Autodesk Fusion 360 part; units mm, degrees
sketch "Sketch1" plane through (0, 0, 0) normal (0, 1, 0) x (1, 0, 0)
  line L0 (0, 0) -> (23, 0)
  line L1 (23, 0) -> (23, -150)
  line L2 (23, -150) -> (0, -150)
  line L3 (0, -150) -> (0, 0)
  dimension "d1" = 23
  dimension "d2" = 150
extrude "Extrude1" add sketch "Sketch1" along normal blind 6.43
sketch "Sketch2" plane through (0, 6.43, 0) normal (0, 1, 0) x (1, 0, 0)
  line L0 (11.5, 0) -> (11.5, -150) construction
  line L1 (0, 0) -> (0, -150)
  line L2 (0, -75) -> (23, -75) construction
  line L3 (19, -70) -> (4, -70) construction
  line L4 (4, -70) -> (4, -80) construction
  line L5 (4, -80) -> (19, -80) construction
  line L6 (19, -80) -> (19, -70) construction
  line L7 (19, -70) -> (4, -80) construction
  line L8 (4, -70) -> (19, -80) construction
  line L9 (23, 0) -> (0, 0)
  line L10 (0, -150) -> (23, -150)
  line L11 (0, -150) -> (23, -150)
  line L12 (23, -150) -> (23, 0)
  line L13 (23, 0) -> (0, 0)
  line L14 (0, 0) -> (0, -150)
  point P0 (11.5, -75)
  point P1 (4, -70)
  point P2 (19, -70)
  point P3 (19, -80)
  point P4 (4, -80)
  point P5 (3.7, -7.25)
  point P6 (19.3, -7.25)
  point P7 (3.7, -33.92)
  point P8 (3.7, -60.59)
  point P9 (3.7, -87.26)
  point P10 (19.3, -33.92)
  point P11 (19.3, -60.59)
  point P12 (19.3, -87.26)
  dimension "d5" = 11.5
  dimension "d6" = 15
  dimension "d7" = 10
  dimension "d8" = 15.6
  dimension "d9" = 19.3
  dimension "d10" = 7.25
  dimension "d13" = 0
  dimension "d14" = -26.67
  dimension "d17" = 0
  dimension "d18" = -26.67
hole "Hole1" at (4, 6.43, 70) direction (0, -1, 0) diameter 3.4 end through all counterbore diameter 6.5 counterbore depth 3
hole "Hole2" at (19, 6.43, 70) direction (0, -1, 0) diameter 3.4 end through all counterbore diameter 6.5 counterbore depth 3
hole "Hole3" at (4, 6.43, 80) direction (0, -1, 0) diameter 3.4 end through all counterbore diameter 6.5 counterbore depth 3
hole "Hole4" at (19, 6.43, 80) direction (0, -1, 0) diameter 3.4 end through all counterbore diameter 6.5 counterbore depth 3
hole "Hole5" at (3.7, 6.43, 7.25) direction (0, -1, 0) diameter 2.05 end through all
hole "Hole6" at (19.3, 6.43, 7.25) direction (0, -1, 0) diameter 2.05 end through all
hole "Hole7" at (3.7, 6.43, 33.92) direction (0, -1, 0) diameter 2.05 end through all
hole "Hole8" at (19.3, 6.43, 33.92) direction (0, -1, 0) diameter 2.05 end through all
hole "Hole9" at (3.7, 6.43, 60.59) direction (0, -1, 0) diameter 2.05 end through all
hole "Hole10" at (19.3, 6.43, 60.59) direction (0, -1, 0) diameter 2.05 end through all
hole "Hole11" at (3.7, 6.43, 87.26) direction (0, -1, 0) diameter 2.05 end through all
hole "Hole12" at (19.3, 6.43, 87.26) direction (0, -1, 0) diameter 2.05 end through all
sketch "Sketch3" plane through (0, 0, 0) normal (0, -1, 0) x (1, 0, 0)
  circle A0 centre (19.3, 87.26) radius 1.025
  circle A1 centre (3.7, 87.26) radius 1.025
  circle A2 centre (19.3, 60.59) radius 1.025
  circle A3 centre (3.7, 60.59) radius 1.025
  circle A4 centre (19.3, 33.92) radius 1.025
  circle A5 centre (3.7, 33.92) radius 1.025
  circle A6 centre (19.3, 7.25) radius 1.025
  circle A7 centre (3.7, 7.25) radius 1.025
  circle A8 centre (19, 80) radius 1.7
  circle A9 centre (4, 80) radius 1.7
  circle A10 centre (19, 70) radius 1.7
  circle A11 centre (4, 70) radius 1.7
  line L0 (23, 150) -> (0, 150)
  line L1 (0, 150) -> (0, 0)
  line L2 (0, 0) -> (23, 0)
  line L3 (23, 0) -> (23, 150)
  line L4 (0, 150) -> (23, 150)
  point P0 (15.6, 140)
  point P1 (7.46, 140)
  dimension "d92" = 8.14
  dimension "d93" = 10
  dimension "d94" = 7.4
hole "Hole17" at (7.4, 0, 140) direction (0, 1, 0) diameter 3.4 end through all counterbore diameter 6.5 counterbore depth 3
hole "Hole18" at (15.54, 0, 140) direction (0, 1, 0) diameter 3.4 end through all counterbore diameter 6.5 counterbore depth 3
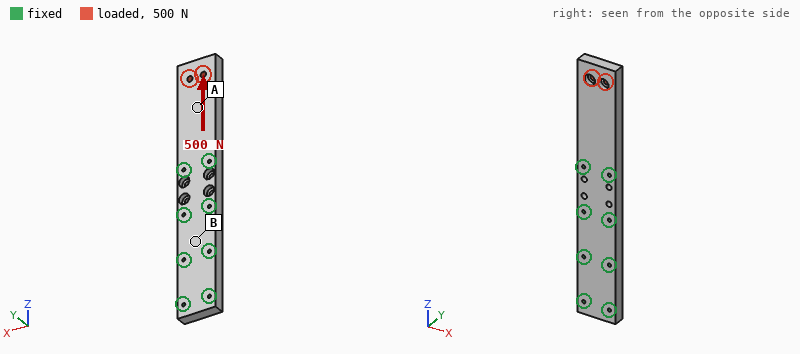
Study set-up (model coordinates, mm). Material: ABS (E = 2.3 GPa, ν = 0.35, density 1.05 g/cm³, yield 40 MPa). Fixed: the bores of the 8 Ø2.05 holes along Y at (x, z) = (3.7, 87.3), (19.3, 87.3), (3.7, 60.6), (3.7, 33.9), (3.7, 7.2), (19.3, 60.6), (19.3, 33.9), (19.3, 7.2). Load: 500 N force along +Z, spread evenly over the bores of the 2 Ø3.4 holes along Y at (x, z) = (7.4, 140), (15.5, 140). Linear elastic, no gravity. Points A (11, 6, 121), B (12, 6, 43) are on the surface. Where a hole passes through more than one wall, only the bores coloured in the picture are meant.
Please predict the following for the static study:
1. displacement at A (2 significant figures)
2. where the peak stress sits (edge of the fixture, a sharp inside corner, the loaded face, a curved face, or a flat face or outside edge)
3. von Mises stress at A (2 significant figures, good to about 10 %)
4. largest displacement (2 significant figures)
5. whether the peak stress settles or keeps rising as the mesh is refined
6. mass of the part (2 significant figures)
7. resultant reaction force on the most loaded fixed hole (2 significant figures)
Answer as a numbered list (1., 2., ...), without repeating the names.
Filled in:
1. 0.42 mm
2. edge of the fixture
3. 8.1 MPa
4. 1.3 mm
5. keeps rising
6. 22 g
7. 230 N
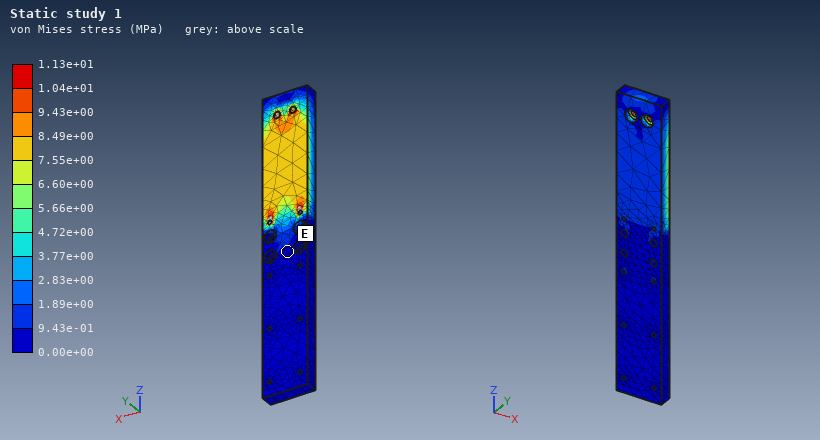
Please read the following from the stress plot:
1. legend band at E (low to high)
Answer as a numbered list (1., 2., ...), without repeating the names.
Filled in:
1. 0.00e+00 to 9.43e-01 MPa
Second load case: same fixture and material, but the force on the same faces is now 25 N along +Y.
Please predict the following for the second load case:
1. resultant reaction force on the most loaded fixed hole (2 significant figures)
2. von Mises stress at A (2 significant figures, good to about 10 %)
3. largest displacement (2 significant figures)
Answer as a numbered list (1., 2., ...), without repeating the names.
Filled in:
1. 19 N
2. 3.0 MPa
3. 1.4 mm
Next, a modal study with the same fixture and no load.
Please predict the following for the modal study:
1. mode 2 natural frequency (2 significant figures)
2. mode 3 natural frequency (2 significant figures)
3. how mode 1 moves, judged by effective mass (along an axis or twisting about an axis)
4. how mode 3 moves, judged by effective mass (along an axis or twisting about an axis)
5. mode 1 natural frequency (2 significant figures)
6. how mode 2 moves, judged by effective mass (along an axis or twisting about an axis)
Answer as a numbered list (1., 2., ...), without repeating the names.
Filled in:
1. 1300 Hz
2. 1900 Hz
3. along Y
4. twisting about Z
5. 390 Hz
6. along X
